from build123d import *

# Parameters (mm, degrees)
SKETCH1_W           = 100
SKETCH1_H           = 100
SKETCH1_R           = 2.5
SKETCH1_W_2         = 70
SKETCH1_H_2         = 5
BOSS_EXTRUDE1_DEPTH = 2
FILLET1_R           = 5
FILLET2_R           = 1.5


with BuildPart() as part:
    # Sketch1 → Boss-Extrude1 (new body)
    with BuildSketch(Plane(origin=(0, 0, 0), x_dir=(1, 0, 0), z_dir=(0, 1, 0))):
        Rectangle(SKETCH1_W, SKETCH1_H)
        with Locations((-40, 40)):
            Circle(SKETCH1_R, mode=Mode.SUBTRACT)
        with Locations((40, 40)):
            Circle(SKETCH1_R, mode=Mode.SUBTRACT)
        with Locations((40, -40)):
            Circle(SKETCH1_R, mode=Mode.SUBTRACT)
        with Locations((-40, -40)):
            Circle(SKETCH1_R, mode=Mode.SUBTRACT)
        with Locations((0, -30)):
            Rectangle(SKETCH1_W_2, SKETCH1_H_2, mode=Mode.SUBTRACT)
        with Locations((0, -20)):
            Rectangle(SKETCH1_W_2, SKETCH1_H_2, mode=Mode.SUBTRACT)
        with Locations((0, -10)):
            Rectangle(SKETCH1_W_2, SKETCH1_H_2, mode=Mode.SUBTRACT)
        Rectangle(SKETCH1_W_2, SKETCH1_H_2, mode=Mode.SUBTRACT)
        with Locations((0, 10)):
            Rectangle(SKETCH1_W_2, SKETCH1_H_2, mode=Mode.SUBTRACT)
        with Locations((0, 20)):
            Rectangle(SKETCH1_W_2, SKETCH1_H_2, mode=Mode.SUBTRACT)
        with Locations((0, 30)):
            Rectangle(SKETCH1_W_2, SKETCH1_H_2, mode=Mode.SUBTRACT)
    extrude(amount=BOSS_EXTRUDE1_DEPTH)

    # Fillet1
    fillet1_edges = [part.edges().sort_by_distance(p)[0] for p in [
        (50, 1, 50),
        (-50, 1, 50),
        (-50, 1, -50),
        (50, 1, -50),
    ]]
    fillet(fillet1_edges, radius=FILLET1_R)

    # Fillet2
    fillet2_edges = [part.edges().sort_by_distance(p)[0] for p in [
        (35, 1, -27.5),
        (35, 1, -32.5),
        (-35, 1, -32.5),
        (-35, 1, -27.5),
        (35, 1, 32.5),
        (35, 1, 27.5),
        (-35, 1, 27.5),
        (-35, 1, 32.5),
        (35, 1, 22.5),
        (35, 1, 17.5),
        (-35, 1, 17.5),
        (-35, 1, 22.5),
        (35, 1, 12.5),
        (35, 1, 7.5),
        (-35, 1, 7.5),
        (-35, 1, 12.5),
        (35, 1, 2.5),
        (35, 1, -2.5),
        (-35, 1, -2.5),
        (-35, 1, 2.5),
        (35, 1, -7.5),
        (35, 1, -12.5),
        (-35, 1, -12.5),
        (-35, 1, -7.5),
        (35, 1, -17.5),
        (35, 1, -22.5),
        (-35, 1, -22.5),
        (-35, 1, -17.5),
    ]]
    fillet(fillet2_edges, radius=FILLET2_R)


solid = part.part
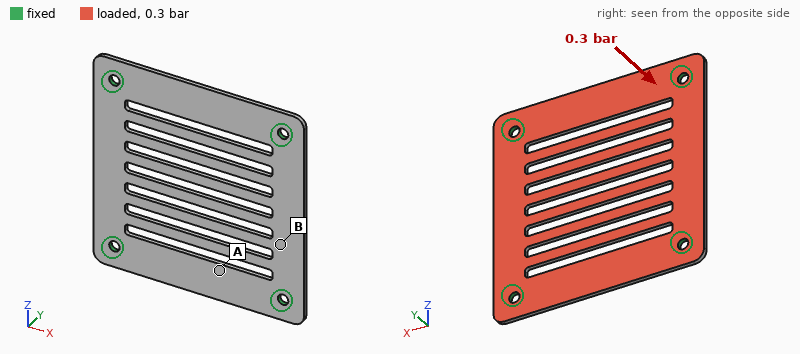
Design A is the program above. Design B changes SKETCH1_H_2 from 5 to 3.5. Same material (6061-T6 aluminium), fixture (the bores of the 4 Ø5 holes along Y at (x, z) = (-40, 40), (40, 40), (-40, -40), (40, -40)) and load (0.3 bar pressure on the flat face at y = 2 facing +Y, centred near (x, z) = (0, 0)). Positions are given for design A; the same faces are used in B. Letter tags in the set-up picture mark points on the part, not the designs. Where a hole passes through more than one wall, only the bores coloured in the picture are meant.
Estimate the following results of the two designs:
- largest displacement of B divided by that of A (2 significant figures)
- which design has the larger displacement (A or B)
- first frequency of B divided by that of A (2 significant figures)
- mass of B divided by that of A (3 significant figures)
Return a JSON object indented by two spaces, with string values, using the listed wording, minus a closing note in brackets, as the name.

{
  "largest displacement of B divided by that of A": "1.1",
  "which design has the larger displacement": "B",
  "first frequency of B divided by that of A": "0.94",
  "mass of B divided by that of A": "1.10"
}
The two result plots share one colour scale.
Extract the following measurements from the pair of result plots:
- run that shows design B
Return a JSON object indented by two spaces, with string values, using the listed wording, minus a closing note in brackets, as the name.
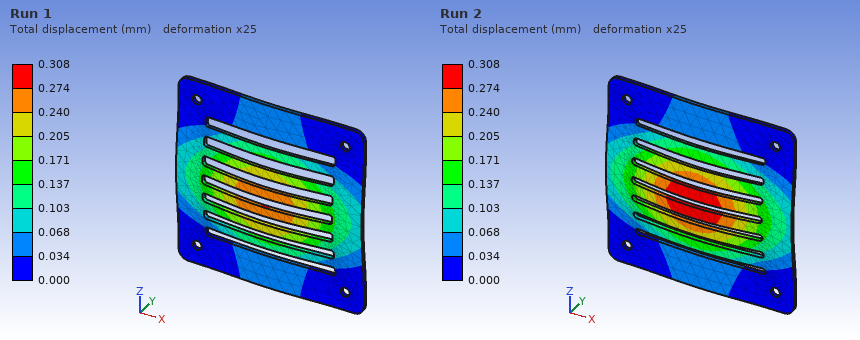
{
  "run that shows design B": "Run 2"
}
